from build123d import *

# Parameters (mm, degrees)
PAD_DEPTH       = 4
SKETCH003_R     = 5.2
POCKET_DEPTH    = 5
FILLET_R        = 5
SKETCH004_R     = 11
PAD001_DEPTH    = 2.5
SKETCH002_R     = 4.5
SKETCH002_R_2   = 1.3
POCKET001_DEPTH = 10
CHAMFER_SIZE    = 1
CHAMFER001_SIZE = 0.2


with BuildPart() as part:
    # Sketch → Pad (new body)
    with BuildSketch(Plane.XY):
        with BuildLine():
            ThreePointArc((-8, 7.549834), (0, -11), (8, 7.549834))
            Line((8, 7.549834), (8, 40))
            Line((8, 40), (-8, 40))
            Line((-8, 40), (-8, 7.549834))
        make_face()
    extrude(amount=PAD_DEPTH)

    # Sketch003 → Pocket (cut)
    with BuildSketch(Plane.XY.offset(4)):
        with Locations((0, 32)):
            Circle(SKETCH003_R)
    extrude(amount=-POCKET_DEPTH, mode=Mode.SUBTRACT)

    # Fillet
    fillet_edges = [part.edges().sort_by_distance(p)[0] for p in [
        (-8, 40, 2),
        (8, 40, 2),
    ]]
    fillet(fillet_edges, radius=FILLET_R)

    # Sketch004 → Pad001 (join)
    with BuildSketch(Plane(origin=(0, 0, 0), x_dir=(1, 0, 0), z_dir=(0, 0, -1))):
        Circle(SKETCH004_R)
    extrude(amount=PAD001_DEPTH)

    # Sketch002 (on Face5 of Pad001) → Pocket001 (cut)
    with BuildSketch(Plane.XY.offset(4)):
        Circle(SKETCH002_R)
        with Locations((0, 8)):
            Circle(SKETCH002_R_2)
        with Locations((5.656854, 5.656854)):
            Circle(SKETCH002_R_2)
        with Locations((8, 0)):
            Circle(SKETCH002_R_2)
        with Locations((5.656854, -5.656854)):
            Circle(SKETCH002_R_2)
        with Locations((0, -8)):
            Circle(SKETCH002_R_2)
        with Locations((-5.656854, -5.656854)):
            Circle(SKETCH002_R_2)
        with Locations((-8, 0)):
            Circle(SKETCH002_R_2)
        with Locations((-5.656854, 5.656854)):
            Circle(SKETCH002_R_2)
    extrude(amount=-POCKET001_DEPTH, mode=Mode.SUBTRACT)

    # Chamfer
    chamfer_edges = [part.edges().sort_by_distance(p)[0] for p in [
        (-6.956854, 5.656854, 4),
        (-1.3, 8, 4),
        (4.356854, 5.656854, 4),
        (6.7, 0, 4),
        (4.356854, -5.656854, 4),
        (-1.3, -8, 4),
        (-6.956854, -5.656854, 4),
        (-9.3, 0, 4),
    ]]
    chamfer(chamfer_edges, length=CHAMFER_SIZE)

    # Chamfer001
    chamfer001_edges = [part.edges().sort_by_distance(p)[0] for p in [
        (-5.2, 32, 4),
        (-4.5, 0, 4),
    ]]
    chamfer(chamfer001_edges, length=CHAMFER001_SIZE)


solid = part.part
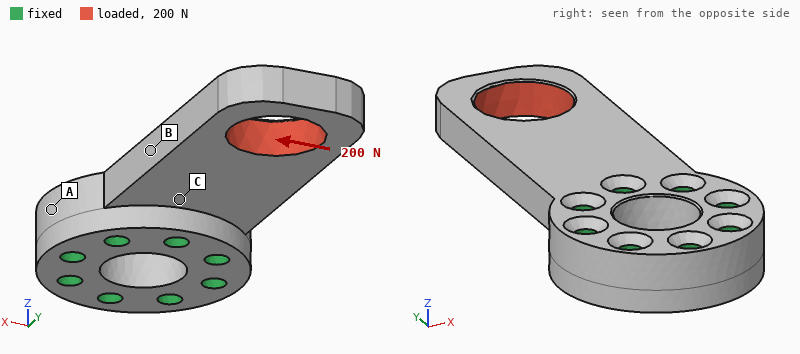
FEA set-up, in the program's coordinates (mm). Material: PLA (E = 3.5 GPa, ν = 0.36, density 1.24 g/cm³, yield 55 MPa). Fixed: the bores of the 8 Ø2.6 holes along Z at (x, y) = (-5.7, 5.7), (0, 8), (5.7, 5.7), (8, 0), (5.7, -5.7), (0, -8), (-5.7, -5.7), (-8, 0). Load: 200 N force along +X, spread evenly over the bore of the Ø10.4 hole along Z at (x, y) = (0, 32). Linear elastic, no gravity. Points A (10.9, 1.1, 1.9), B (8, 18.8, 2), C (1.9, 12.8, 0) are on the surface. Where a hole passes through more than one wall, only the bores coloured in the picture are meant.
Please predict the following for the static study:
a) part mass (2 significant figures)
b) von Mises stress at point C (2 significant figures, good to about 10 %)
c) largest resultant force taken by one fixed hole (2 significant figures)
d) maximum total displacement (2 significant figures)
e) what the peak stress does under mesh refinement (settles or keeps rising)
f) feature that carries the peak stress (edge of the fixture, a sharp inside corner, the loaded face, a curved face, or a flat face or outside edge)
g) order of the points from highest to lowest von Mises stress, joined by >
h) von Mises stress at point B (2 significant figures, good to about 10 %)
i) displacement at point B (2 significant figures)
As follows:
4.1 g
12 MPa
340 N
0.56 mm
keeps rising
edge of the fixture
B > C > A
16 MPa
0.13 mm
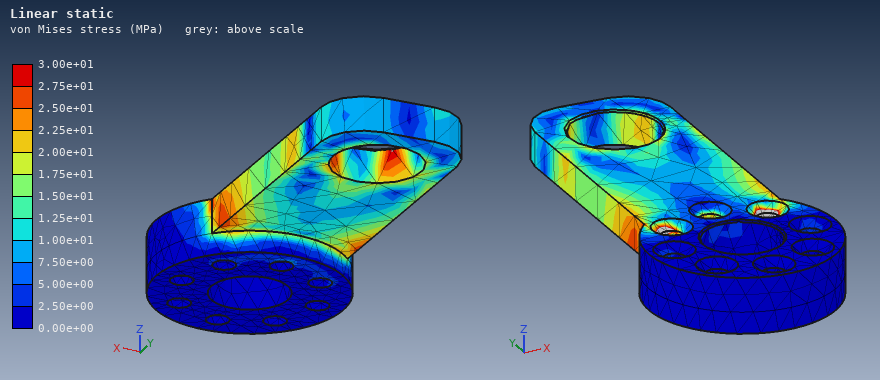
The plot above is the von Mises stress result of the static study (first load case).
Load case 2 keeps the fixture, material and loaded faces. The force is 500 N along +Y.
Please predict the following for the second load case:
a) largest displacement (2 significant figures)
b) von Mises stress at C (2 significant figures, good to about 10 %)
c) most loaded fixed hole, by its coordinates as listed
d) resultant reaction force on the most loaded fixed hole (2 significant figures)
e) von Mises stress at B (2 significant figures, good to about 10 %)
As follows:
0.15 mm
9.5 MPa
(0, 8)
200 N
10.0 MPa
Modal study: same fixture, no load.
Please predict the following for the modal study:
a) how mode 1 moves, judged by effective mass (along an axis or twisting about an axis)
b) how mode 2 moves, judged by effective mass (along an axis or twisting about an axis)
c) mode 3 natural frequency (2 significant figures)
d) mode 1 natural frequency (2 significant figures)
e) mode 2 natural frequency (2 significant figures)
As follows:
along Z
along X
4000 Hz
1400 Hz
3800 Hz
